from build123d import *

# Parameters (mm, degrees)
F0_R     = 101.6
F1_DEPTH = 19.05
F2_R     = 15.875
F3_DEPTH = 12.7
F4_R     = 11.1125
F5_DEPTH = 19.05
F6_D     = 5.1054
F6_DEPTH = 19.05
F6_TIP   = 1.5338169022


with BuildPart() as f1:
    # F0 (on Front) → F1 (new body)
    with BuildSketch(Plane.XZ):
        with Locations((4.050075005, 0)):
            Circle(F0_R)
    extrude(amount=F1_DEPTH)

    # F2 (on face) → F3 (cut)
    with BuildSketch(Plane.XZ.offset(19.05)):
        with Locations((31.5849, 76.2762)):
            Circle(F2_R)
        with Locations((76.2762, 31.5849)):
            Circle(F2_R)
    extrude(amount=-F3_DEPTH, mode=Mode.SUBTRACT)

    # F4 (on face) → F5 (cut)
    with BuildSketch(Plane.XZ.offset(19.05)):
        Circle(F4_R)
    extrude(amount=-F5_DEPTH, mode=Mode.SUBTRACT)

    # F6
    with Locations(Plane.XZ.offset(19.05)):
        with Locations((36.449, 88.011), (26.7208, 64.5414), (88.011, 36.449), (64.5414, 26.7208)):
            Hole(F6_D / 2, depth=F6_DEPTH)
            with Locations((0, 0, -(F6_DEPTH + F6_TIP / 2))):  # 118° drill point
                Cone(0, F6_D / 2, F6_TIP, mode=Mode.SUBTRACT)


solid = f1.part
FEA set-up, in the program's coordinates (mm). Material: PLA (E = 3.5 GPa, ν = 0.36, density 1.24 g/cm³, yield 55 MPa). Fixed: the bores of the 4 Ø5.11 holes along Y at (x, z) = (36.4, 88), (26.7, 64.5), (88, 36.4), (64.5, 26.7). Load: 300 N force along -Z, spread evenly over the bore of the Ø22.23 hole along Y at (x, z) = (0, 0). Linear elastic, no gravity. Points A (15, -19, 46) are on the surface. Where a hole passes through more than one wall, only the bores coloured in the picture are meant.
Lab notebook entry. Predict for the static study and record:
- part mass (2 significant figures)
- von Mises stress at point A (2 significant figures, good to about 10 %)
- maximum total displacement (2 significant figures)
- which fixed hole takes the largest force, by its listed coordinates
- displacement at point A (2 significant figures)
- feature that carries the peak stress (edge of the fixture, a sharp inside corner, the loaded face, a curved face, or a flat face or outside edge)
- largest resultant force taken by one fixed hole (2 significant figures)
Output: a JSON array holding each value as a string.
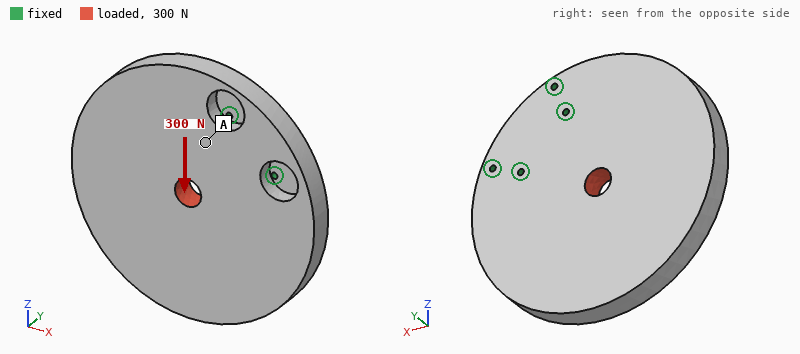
["730 g", "0.19 MPa", "53 µm", "(26.7, 64.5)", "14 µm", "edge of the fixture", "230 N"]
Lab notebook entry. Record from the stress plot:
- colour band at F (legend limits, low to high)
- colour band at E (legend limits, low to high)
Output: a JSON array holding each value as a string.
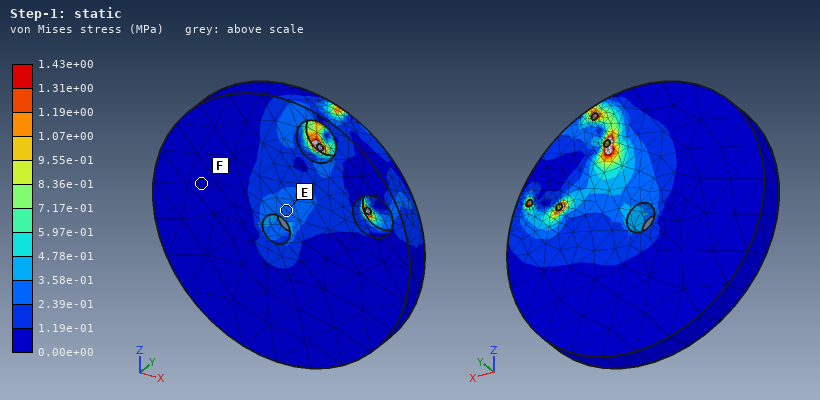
["0.00e+00 to 1.19e-01 MPa", "2.39e-01 to 3.58e-01 MPa"]
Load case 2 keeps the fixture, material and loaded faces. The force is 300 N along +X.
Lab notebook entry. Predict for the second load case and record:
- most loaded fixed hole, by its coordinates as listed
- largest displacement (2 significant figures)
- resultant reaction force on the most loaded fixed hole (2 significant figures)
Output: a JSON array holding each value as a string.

["(64.5, 26.7)", "53 µm", "220 N"]
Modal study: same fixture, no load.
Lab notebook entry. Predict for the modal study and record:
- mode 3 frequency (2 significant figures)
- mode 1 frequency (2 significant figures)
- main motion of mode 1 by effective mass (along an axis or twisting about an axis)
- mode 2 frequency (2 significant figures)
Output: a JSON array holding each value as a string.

["520 Hz", "140 Hz", "along Y", "300 Hz"]
